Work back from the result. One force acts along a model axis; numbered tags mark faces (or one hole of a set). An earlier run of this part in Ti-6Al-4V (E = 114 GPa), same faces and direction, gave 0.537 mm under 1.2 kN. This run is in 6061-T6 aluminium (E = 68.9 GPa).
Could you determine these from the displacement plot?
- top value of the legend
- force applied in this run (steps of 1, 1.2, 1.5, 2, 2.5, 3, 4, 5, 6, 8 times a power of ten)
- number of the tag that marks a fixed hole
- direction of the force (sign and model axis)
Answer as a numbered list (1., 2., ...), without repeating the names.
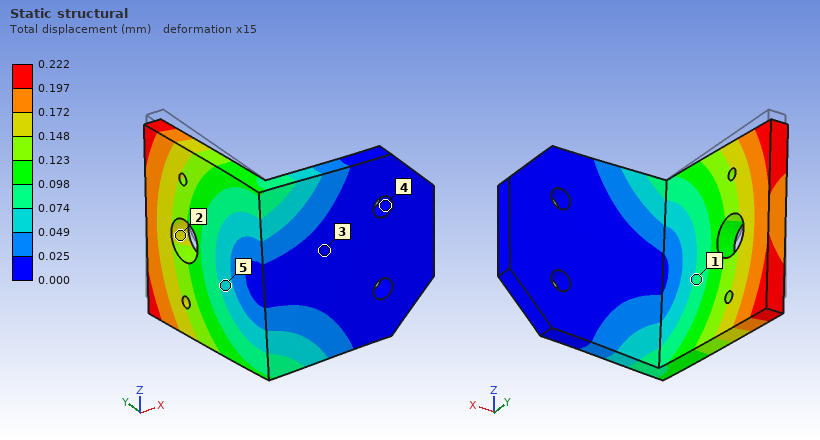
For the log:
1. 0.222 mm
2. 300 N
3. 4
4. -Z
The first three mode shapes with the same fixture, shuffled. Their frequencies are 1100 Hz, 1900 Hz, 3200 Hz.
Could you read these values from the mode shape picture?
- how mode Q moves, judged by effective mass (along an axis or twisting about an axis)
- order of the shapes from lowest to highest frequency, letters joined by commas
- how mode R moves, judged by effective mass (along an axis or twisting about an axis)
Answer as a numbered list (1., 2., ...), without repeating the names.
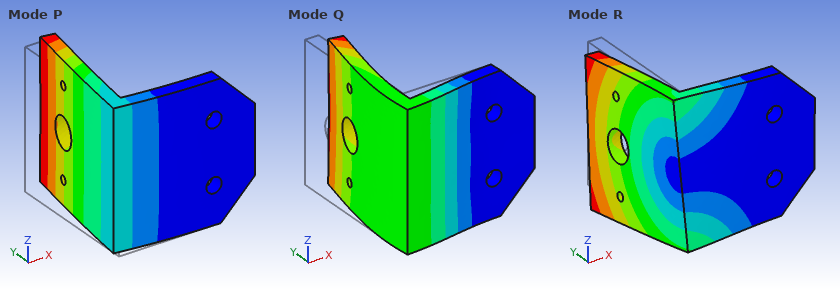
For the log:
1. along Y
2. P, R, Q
3. along Z
